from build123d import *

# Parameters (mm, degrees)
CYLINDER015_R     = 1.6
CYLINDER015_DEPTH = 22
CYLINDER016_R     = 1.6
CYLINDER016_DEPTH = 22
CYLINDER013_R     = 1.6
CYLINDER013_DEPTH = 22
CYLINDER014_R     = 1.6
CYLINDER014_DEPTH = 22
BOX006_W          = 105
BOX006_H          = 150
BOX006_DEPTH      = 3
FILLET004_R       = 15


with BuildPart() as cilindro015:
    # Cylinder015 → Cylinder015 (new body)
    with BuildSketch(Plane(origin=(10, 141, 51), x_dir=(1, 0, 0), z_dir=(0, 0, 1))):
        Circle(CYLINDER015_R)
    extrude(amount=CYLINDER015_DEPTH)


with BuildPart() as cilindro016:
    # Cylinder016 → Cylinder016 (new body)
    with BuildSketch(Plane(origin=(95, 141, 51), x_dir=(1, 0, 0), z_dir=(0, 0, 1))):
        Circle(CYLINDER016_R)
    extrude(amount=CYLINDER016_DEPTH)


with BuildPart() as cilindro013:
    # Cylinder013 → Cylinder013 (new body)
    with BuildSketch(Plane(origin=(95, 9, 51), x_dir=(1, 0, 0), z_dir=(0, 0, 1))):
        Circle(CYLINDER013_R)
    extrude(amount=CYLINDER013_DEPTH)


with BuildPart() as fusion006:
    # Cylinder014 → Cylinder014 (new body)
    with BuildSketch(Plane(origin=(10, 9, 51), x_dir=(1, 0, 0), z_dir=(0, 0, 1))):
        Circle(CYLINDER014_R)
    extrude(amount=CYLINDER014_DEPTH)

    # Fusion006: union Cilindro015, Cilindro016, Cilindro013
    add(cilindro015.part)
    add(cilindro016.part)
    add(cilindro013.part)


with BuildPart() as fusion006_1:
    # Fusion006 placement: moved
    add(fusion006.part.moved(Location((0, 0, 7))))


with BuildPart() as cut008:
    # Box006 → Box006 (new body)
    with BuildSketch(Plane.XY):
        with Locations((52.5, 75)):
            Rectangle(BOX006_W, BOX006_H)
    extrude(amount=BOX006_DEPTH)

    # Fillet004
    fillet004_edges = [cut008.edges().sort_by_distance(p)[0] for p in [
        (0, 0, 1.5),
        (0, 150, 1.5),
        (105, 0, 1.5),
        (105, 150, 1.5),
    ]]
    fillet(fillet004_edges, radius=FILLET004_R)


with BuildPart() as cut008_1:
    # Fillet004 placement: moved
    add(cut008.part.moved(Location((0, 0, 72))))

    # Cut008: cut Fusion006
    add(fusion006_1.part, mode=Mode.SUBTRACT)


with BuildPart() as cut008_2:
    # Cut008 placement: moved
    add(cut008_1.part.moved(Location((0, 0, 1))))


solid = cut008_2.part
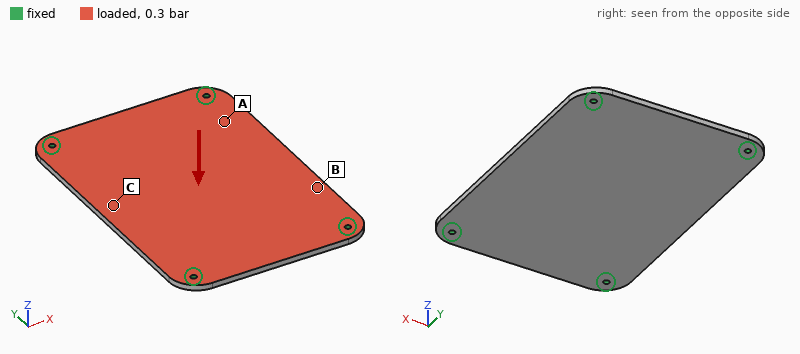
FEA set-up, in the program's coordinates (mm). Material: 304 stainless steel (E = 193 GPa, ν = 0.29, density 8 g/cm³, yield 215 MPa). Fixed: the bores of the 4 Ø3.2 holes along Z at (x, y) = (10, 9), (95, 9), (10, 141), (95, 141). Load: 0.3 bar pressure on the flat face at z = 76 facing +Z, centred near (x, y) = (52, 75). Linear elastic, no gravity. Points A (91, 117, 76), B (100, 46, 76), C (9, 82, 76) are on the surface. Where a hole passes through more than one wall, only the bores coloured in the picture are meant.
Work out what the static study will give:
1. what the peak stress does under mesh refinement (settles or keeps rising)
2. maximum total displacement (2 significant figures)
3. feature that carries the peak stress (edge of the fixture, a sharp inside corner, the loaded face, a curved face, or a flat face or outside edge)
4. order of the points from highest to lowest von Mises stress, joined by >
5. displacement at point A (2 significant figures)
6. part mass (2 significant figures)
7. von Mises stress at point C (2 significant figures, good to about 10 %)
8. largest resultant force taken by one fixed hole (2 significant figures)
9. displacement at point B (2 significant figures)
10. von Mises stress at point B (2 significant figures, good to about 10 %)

keeps rising
90 µm
edge of the fixture
C > B > A
35 µm
370 g
19 MPa
120 N
54 µm
11 MPa
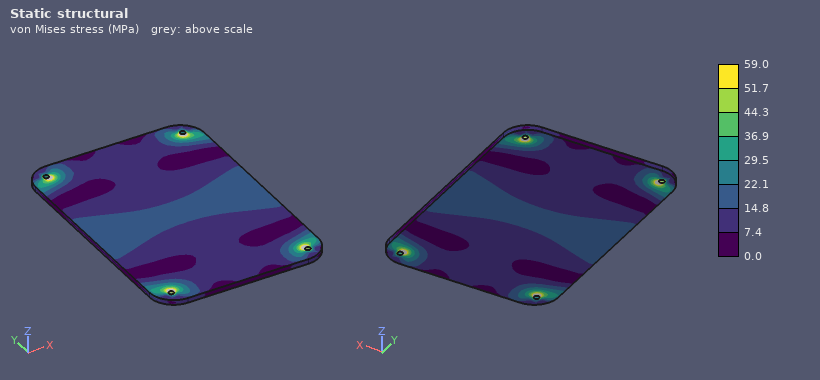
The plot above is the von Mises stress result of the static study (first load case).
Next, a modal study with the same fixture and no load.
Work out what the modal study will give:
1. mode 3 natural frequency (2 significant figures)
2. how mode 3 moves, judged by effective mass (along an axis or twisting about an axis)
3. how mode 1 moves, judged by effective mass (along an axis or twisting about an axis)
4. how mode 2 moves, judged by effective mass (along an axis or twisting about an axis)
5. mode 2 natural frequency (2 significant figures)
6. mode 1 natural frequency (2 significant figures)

1700 Hz
twisting about X
along Z
twisting about Y
1100 Hz
690 Hz
